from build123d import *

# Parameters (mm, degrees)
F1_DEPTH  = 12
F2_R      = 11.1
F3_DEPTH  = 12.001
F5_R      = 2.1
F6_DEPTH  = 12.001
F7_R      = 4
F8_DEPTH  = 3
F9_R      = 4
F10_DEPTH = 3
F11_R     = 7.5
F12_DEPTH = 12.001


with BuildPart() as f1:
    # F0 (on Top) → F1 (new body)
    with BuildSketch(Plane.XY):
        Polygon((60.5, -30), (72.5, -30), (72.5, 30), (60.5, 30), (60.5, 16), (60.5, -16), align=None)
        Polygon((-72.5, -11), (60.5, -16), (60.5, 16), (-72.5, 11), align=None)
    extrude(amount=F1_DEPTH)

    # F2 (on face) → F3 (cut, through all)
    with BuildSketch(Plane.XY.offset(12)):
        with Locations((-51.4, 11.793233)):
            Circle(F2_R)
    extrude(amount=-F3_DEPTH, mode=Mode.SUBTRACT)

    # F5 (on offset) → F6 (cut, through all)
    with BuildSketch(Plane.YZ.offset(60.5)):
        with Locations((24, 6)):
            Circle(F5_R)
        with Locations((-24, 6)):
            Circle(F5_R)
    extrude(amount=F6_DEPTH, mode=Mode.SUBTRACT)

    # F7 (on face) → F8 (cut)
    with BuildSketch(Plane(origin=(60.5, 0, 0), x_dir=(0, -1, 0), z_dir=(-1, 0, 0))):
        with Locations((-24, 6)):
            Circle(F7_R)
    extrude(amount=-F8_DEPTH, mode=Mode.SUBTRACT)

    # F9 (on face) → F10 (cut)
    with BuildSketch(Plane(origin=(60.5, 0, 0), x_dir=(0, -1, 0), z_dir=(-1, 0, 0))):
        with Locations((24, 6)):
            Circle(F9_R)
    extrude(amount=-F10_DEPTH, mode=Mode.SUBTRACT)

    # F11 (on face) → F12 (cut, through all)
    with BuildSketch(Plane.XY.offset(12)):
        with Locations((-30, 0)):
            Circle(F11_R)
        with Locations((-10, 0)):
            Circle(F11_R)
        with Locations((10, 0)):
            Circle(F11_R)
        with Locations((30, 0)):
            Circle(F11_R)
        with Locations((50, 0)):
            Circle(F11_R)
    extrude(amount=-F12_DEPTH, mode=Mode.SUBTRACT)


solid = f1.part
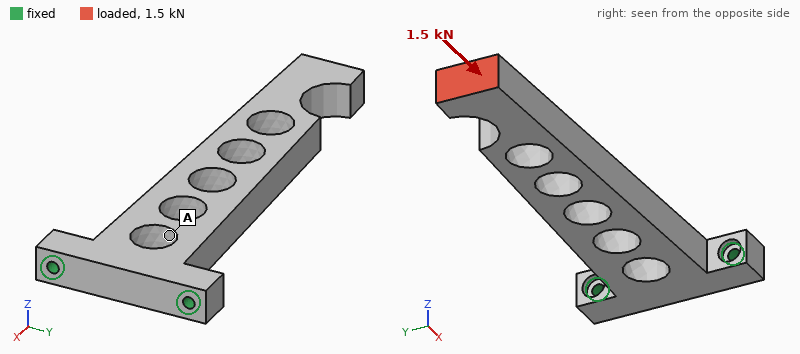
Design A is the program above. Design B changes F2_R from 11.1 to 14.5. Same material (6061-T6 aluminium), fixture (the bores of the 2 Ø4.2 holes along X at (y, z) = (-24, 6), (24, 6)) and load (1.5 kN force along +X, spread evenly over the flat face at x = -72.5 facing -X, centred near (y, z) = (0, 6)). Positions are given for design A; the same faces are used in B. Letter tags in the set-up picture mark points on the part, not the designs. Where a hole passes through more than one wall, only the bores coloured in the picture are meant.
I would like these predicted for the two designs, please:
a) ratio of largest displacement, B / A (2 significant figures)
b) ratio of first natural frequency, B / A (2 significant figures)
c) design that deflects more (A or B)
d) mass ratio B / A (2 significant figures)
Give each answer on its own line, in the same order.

2.9
1.1
B
0.96
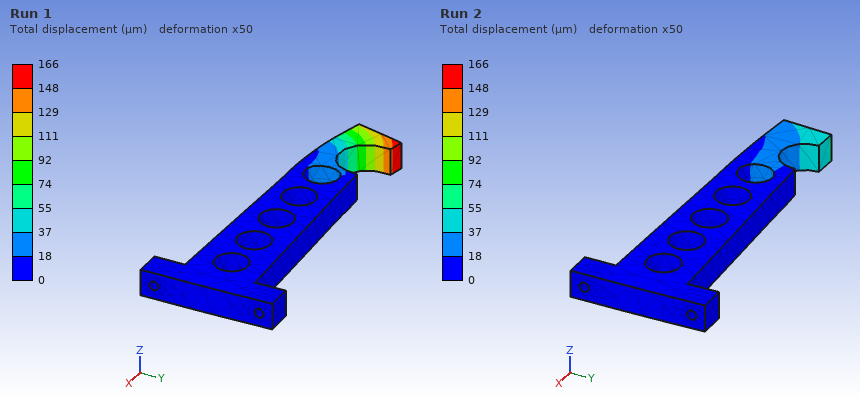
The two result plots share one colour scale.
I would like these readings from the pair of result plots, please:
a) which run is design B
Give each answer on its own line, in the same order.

Run 1
